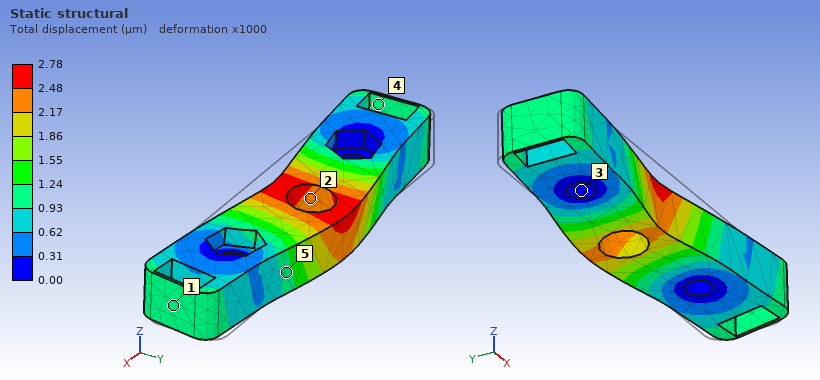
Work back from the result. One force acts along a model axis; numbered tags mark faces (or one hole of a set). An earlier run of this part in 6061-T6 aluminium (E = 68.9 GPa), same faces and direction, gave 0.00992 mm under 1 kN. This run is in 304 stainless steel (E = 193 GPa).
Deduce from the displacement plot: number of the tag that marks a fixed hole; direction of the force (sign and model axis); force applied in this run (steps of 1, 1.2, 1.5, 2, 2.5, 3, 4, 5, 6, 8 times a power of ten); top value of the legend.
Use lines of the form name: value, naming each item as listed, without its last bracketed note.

number of the tag that marks a fixed hole: 3
direction of the force: +Y
force applied in this run: 800 N
top value of the legend: 2.78 µm
